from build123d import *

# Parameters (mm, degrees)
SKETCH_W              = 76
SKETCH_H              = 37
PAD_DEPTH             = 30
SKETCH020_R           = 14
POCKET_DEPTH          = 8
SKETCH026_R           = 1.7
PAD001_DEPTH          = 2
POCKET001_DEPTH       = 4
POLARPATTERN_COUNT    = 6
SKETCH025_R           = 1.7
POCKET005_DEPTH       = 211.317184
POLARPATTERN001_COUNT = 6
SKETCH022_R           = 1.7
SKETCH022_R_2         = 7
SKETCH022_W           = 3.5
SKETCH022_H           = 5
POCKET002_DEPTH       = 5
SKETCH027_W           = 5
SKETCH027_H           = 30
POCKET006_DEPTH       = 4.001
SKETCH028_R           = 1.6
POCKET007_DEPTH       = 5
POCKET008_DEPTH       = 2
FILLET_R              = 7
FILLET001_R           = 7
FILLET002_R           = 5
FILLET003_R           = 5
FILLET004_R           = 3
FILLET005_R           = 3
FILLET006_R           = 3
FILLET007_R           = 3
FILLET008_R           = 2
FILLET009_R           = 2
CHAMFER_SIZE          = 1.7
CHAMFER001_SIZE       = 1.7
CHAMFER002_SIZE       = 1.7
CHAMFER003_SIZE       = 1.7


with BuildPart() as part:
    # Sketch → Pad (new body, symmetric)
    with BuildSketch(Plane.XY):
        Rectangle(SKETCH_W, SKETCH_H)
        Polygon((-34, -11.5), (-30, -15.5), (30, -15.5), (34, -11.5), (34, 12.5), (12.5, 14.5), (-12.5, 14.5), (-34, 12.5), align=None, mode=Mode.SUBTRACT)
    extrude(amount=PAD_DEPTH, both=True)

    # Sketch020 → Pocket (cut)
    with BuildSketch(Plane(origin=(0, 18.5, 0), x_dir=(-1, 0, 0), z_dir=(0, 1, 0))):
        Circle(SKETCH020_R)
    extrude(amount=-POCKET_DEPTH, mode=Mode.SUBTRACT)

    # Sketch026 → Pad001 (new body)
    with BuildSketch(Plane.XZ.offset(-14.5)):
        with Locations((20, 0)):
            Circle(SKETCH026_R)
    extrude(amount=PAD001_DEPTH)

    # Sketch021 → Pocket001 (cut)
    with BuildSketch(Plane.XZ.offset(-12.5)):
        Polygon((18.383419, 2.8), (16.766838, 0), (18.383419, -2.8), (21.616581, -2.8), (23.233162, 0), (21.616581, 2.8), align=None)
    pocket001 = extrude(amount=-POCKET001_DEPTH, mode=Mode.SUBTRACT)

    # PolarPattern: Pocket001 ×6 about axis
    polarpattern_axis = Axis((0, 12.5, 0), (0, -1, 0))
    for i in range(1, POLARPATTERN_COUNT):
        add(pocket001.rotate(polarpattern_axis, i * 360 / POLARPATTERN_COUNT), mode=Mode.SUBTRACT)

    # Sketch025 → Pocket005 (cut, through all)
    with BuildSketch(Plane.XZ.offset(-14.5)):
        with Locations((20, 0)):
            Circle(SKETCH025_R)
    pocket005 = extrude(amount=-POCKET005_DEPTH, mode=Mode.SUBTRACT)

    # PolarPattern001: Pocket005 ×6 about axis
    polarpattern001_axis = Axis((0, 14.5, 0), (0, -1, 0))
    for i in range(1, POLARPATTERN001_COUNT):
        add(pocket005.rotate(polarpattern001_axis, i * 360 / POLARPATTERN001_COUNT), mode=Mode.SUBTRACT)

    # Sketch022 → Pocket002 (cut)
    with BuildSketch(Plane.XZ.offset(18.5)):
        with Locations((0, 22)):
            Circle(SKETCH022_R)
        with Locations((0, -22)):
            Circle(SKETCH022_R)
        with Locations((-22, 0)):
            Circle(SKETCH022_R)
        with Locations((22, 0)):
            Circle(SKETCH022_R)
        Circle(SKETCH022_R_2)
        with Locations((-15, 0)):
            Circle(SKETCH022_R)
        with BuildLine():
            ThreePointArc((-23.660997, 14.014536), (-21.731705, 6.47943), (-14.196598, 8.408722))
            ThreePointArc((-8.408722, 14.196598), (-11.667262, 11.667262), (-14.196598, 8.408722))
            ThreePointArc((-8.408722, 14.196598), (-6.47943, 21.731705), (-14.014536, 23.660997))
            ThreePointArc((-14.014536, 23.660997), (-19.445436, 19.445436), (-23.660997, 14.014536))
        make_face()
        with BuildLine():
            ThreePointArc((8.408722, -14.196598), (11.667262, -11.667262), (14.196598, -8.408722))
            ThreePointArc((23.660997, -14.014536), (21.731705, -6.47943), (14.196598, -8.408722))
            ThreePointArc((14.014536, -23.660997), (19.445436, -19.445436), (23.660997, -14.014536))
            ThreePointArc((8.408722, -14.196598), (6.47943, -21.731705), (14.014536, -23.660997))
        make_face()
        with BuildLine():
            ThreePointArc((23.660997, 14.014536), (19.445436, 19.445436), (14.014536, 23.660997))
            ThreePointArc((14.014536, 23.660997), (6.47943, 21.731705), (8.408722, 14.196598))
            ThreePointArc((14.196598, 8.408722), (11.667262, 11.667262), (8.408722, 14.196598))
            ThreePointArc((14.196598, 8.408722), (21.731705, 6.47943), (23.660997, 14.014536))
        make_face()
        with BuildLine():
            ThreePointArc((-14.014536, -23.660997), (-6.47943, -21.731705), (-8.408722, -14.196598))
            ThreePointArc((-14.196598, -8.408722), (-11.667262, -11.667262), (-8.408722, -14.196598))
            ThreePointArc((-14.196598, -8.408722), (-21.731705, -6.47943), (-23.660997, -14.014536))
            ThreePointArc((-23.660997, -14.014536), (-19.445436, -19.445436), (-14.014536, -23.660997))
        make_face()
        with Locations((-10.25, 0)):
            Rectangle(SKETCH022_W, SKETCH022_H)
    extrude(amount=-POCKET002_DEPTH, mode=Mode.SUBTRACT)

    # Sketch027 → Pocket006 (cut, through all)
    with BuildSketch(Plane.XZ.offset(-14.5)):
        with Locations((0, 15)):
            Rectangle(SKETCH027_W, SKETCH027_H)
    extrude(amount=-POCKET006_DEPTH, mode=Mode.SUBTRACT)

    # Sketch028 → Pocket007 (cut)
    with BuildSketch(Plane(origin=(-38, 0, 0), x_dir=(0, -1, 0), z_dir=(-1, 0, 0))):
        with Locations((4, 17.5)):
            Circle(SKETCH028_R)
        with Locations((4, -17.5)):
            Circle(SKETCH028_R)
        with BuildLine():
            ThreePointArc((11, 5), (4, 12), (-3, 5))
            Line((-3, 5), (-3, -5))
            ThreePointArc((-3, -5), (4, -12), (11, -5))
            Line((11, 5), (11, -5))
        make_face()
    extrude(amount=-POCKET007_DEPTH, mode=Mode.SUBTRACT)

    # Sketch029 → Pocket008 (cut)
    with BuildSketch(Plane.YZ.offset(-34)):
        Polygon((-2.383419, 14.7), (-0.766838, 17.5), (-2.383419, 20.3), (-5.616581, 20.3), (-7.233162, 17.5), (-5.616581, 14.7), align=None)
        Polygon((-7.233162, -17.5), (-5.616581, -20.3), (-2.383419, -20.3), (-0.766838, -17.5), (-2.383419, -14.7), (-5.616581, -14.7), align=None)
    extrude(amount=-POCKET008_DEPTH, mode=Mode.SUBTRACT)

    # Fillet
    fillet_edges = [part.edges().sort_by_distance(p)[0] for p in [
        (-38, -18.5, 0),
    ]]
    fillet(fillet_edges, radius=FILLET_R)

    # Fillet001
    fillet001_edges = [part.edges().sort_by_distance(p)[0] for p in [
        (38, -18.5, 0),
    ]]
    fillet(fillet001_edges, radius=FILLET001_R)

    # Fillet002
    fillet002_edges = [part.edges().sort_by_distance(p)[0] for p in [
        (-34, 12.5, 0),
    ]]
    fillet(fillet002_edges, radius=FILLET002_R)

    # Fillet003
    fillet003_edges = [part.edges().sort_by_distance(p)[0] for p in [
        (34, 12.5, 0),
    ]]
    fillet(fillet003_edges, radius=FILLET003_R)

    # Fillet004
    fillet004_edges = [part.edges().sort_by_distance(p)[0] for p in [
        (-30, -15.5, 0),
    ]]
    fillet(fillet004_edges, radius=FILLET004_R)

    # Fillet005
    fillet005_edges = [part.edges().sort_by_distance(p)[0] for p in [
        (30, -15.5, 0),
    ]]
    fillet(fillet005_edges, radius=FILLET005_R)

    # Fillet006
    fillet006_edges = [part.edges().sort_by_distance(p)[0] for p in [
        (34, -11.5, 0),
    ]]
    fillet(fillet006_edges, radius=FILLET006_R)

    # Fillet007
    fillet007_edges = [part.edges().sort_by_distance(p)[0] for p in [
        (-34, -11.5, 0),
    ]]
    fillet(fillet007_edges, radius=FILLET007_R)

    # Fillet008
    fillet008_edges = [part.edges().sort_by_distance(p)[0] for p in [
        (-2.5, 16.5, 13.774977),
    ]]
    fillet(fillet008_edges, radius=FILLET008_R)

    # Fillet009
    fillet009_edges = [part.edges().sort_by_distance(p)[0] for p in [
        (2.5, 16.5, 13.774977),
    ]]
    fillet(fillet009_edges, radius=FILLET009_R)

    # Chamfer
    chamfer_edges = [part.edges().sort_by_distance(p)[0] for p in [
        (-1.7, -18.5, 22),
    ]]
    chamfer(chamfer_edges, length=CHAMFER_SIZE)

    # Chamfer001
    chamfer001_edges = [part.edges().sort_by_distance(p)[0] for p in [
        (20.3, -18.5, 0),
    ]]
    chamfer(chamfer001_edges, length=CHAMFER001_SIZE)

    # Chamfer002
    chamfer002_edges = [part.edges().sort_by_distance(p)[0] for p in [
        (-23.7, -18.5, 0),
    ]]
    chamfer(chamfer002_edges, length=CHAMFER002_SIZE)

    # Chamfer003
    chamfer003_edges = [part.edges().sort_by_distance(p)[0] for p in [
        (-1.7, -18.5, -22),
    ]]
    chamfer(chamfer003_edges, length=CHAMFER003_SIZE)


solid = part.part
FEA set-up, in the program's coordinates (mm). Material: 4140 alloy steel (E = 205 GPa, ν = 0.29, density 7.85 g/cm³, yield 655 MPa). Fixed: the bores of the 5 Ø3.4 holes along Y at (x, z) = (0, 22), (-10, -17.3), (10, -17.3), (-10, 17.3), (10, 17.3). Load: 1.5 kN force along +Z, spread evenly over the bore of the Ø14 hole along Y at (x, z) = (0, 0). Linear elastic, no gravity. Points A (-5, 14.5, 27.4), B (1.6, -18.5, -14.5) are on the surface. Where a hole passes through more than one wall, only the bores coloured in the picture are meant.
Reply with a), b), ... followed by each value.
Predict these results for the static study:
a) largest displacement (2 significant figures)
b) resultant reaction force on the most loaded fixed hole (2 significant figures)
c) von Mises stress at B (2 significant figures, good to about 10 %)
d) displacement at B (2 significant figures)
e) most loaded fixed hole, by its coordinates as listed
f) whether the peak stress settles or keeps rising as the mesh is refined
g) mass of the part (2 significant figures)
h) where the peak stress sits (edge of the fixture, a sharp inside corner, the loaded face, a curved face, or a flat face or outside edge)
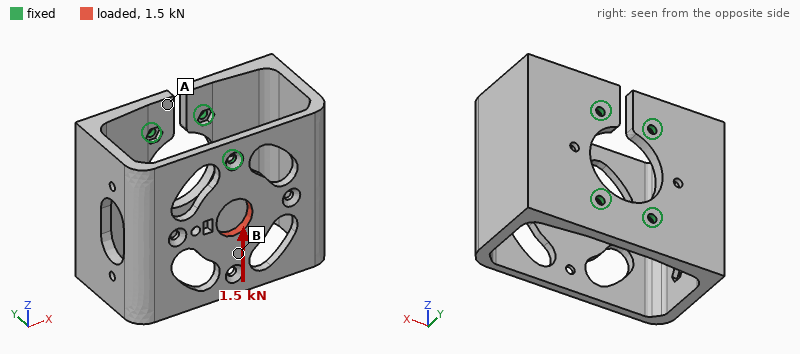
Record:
a) 8.8 µm
b) 1.4 kN
c) 11 MPa
d) 8.4 µm
e) (0, 22)
f) keeps rising
g) 320 g
h) edge of the fixture
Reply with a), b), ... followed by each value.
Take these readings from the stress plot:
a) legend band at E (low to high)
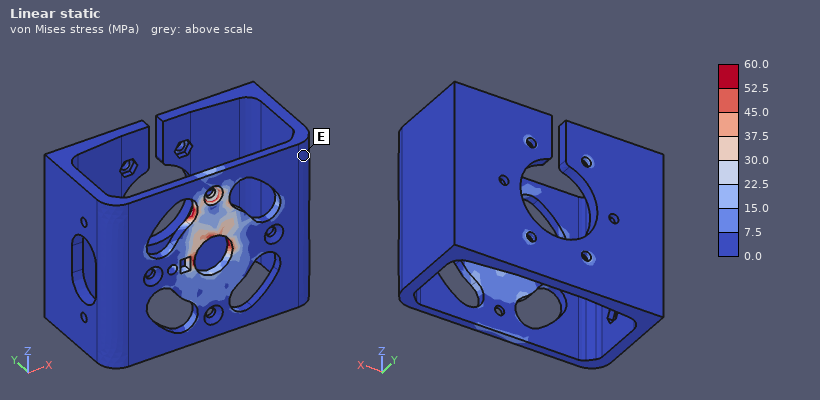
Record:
a) 0.0 to 7.5 MPa
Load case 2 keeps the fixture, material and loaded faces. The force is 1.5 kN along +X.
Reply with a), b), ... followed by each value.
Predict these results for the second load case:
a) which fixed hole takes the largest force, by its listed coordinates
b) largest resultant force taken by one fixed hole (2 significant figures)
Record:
a) (0, 22)
b) 1.4 kN
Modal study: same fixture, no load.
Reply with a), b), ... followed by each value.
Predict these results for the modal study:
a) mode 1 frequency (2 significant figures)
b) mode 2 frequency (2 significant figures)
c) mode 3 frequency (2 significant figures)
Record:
a) 2100 Hz
b) 2100 Hz
c) 2900 Hz
